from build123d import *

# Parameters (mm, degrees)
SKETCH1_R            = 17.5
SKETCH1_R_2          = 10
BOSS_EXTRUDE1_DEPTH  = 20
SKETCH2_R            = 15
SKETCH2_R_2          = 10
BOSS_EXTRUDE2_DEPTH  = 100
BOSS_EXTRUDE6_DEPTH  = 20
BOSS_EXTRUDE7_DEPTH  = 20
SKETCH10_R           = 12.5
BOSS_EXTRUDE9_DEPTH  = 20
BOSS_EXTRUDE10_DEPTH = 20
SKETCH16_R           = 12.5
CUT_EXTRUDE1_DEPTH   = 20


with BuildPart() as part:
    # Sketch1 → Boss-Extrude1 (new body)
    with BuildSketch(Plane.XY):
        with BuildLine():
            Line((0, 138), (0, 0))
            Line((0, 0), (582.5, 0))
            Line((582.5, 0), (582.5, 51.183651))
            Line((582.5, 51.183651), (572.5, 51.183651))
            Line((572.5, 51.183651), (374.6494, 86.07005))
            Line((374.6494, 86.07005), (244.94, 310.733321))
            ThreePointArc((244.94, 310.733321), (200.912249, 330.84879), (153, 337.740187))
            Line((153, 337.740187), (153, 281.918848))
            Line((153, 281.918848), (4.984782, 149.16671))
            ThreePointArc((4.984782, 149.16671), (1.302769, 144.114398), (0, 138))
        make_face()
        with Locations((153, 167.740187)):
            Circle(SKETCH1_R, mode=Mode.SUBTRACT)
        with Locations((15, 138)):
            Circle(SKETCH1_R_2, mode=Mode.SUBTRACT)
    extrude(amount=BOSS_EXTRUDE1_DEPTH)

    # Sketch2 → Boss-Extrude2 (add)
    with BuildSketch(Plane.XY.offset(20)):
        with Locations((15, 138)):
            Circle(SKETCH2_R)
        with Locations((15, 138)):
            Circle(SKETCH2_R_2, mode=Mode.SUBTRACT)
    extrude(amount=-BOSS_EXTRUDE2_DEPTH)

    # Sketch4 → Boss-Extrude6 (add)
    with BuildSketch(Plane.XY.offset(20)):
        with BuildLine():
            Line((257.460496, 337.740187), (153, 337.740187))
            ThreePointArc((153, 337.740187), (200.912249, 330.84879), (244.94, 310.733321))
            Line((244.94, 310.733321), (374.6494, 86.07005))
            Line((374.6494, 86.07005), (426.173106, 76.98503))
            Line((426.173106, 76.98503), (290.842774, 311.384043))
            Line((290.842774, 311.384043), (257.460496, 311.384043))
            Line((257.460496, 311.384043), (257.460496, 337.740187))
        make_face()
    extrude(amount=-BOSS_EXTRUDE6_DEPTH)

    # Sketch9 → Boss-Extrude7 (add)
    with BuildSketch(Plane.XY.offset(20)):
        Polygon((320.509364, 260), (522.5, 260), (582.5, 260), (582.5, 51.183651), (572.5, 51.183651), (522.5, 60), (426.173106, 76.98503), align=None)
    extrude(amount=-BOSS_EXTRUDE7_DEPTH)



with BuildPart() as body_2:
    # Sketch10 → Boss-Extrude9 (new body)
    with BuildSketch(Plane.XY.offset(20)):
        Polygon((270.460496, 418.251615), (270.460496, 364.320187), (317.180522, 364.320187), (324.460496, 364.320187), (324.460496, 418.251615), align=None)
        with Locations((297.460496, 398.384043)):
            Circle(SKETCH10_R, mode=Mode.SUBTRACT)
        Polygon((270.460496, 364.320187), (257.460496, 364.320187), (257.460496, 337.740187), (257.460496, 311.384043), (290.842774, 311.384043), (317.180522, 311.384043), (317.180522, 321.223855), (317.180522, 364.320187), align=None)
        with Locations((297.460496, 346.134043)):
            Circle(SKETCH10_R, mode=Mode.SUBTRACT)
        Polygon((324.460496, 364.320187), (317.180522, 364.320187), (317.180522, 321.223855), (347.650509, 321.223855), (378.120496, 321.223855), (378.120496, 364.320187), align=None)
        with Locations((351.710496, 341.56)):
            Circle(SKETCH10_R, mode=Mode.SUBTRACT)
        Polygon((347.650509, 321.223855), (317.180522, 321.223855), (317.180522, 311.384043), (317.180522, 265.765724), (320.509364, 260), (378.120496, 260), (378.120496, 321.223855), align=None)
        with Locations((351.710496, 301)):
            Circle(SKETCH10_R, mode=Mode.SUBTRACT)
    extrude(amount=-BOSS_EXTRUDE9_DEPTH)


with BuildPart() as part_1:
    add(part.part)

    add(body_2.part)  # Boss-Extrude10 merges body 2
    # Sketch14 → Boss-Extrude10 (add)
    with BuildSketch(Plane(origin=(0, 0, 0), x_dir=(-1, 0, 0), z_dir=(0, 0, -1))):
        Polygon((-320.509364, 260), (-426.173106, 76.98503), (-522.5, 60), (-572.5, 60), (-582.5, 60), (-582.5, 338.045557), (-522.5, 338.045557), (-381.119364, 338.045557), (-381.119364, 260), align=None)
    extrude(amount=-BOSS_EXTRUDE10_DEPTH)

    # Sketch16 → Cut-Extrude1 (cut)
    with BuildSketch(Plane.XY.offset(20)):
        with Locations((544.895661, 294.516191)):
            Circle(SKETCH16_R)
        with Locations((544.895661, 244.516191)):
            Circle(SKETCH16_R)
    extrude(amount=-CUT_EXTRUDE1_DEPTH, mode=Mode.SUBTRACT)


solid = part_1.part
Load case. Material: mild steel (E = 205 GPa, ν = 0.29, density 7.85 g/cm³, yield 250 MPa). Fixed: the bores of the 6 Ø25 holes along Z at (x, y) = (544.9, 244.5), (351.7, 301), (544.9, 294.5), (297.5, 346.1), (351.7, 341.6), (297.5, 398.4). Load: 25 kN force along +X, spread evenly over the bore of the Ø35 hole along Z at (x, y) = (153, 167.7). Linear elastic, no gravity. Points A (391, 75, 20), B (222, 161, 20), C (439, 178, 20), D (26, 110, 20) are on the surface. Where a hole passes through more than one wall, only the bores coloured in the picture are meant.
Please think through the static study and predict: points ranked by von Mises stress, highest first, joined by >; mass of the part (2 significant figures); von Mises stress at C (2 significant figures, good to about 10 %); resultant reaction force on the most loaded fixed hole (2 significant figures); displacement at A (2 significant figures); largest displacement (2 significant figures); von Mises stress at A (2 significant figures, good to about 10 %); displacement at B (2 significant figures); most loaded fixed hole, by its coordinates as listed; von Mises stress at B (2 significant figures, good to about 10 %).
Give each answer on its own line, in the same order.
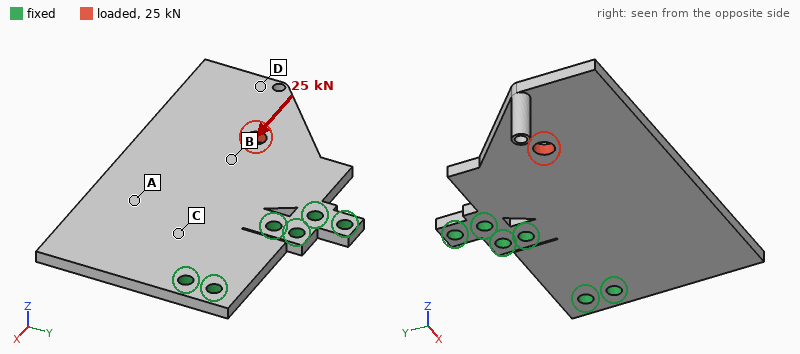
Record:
B > C > A > D
28 kg
6.1 MPa
15 kN
12 µm
21 µm
3.2 MPa
14 µm
(544.9, 244.5)
8.2 MPa
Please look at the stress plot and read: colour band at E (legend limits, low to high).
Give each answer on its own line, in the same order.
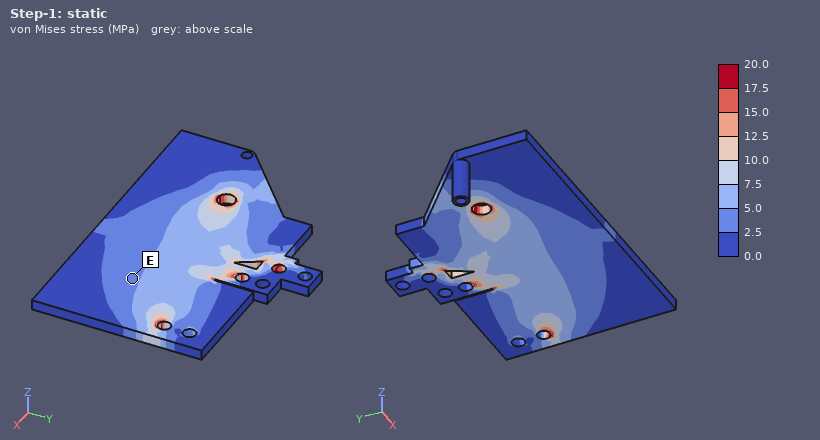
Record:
2.5 to 5.0 MPa
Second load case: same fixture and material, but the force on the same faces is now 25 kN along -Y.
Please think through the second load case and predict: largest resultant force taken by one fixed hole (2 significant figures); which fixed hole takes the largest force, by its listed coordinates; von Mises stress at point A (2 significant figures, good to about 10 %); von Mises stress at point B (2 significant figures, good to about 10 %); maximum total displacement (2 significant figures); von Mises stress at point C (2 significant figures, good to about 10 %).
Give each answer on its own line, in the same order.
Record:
22 kN
(297.5, 346.1)
4.1 MPa
7.9 MPa
43 µm
5.7 MPa
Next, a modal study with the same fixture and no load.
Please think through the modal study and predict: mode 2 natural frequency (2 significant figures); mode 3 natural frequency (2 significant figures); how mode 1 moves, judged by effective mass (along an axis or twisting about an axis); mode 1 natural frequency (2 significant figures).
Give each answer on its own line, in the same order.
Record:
250 Hz
500 Hz
along Z
100 Hz
